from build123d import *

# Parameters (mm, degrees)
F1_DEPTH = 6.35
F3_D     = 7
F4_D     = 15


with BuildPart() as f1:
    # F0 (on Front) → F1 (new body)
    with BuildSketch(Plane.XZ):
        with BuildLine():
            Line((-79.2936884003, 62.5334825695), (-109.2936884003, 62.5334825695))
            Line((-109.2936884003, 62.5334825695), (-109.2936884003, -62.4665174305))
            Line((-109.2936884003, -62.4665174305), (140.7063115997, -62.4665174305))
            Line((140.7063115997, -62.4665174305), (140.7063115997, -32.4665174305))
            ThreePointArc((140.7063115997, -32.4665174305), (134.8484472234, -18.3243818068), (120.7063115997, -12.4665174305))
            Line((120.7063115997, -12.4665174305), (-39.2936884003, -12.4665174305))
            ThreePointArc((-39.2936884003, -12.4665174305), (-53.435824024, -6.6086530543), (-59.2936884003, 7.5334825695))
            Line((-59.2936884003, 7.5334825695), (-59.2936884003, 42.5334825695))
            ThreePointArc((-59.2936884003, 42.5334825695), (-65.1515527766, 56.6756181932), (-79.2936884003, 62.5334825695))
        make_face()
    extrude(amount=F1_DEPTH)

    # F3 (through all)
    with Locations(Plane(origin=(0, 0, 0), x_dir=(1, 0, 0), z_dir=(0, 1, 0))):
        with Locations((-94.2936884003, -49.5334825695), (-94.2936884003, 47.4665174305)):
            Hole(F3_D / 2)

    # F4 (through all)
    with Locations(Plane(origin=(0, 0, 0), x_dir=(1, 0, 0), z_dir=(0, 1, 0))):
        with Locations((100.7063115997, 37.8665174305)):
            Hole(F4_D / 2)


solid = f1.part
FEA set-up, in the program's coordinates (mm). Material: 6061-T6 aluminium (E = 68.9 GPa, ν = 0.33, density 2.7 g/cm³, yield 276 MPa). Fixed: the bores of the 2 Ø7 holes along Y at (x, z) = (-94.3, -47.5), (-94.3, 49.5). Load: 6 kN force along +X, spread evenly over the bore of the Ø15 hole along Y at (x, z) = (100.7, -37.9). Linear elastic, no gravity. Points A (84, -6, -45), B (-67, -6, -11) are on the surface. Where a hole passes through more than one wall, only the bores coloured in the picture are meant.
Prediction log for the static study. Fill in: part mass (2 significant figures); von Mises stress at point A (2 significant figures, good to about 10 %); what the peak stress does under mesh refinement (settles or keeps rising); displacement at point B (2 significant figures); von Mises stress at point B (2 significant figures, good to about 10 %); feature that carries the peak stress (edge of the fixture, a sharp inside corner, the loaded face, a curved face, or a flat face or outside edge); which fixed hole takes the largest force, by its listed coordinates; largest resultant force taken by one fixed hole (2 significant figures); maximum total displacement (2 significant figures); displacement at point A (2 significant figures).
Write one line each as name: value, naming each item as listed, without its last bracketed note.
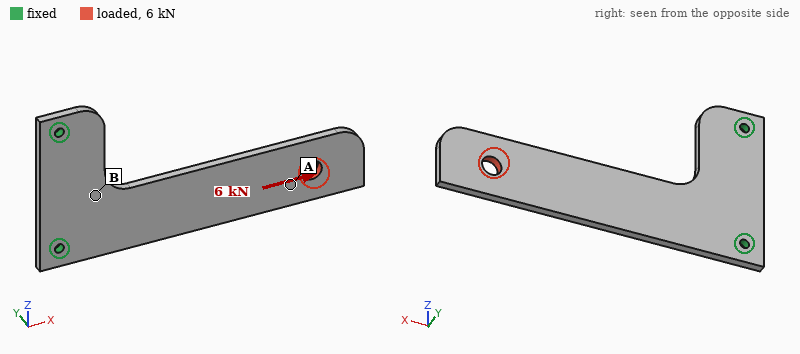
part mass: 270 g
von Mises stress at point A: 23 MPa
what the peak stress does under mesh refinement: keeps rising
displacement at point B: 12 µm
von Mises stress at point B: 6.4 MPa
feature that carries the peak stress: edge of the fixture
which fixed hole takes the largest force, by its listed coordinates: (-94.3, -47.5)
largest resultant force taken by one fixed hole: 5.4 kN
maximum total displacement: 66 µm
displacement at point A: 56 µm
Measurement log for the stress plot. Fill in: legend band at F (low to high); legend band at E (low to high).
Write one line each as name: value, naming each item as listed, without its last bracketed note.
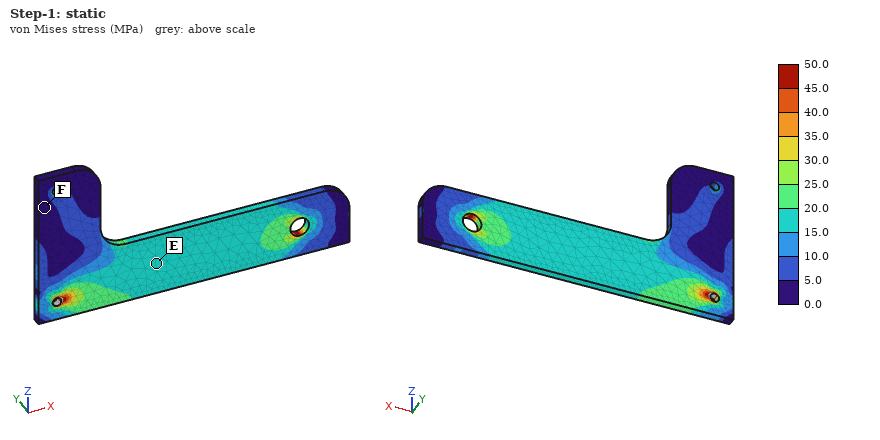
legend band at F: 0.0 to 5.0 MPa
legend band at E: 15.0 to 20.0 MPa
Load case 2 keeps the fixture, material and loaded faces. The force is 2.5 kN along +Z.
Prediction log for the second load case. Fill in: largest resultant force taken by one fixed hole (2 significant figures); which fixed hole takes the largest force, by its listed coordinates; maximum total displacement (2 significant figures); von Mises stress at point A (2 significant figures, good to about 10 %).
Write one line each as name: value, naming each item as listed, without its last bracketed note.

largest resultant force taken by one fixed hole: 6.6 kN
which fixed hole takes the largest force, by its listed coordinates: (-94.3, 49.5)
maximum total displacement: 1.5 mm
von Mises stress at point A: 18 MPa
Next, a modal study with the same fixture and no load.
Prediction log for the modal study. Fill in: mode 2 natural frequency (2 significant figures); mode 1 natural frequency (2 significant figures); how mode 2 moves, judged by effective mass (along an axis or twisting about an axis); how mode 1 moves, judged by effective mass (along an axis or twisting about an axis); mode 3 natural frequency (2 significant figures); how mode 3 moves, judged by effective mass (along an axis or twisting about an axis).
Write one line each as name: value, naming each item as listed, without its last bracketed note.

mode 2 natural frequency: 610 Hz
mode 1 natural frequency: 100 Hz
how mode 2 moves, judged by effective mass: along Y
how mode 1 moves, judged by effective mass: along Y
mode 3 natural frequency: 830 Hz
how mode 3 moves, judged by effective mass: along Z
